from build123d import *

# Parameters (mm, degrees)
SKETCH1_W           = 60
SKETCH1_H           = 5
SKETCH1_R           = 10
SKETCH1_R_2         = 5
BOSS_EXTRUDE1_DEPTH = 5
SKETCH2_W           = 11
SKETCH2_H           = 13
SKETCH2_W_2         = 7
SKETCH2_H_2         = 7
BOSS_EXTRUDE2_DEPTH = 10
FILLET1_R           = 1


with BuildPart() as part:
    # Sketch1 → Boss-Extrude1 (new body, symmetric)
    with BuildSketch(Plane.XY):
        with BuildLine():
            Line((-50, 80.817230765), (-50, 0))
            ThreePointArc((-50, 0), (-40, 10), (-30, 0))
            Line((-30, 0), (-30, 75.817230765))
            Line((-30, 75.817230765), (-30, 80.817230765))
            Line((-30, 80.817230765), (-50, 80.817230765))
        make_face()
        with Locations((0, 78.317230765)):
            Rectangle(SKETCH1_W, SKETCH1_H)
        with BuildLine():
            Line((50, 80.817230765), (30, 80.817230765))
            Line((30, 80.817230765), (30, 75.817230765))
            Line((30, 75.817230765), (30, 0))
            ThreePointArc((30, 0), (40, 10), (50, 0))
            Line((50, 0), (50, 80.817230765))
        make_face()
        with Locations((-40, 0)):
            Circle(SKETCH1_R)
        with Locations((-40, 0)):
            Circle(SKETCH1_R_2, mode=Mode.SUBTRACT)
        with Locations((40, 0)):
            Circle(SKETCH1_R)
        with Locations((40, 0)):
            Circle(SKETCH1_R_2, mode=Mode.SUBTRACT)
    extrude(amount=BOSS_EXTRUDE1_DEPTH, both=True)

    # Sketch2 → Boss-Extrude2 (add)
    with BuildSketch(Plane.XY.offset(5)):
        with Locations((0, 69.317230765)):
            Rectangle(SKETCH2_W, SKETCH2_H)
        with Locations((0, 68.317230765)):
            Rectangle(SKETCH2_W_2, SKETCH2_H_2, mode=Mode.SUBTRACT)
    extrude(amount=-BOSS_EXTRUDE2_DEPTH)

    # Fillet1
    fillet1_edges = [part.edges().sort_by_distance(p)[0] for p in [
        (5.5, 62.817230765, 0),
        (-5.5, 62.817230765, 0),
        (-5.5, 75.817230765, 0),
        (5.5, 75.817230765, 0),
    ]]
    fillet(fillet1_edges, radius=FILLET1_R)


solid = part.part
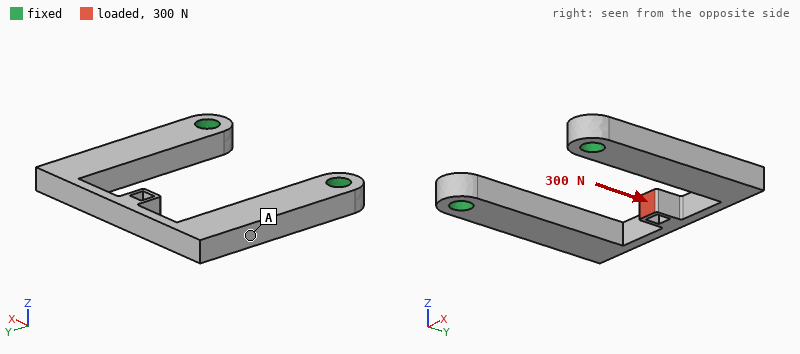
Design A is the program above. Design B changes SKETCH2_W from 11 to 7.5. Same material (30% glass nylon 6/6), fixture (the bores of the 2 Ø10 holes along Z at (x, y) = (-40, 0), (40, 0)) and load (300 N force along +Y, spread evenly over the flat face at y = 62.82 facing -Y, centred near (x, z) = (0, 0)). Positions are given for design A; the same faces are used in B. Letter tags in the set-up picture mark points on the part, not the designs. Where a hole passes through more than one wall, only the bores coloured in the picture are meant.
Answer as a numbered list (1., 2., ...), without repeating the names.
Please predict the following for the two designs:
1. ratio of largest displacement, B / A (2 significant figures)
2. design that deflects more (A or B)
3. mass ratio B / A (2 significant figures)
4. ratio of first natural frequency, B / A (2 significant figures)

1. 1.3
2. B
3. 0.99
4. 1.0
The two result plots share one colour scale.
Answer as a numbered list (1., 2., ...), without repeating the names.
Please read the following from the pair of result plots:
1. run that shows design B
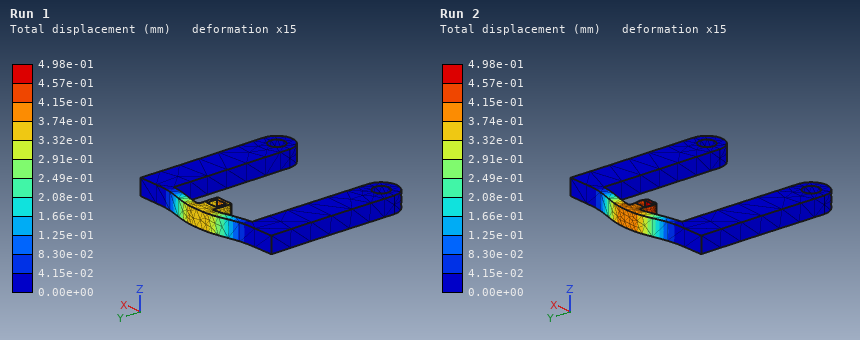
1. Run 2
